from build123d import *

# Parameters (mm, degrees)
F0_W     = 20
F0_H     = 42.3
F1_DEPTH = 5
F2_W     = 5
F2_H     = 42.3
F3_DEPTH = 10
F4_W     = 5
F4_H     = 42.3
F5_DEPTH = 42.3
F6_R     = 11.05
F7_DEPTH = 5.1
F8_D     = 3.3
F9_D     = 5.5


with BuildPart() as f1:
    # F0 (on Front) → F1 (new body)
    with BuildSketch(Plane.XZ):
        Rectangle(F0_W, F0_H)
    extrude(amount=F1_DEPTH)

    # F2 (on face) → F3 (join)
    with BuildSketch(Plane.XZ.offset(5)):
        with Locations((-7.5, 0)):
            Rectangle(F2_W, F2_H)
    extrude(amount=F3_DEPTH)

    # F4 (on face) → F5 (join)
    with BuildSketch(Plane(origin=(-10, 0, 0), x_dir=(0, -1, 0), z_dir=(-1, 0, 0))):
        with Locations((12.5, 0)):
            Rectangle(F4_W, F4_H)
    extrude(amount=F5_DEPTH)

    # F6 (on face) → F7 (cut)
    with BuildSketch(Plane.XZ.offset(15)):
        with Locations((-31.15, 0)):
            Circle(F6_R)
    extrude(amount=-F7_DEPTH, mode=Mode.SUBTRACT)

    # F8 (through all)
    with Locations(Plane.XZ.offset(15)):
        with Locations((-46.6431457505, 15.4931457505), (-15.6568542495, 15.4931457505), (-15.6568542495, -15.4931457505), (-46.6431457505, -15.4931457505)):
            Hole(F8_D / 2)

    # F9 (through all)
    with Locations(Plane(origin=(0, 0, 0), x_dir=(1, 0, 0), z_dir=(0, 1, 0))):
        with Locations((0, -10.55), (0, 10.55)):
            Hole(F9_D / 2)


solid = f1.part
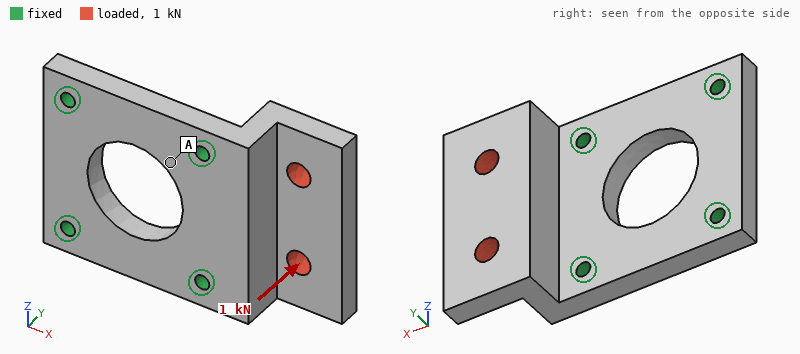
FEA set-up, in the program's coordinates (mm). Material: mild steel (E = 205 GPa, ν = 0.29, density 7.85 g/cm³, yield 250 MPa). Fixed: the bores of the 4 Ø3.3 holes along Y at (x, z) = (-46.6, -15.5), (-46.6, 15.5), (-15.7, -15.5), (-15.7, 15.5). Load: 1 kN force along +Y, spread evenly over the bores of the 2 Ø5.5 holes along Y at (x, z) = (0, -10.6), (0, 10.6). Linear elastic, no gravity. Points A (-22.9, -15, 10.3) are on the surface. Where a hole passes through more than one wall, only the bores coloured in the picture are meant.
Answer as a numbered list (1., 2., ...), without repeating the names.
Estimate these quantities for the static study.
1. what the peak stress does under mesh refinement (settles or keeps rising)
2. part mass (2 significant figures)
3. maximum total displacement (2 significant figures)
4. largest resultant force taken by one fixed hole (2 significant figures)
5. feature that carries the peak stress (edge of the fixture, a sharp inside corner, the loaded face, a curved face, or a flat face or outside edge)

1. keeps rising
2. 100 g
3. 51 µm
4. 550 N
5. edge of the fixture
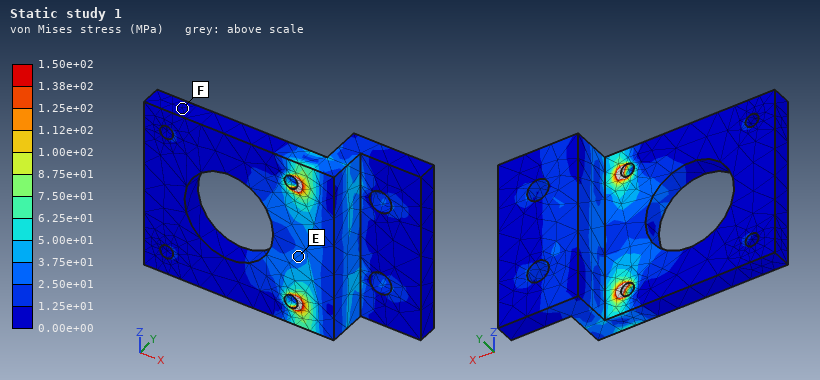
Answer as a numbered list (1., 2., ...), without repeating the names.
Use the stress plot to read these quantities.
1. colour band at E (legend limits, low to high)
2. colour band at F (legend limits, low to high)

1. 2.50e+01 to 3.75e+01 MPa
2. 0.00e+00 to 1.25e+01 MPa
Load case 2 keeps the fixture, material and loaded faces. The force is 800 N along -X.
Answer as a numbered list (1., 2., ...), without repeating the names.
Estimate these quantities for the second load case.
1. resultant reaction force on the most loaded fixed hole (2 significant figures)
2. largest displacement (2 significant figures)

1. 380 N
2. 28 µm
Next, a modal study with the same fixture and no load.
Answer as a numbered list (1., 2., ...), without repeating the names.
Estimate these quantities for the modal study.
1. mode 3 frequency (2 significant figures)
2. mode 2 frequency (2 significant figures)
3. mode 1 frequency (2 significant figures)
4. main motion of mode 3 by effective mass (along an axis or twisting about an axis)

1. 15 kHz
2. 8900 Hz
3. 4200 Hz
4. along Z
